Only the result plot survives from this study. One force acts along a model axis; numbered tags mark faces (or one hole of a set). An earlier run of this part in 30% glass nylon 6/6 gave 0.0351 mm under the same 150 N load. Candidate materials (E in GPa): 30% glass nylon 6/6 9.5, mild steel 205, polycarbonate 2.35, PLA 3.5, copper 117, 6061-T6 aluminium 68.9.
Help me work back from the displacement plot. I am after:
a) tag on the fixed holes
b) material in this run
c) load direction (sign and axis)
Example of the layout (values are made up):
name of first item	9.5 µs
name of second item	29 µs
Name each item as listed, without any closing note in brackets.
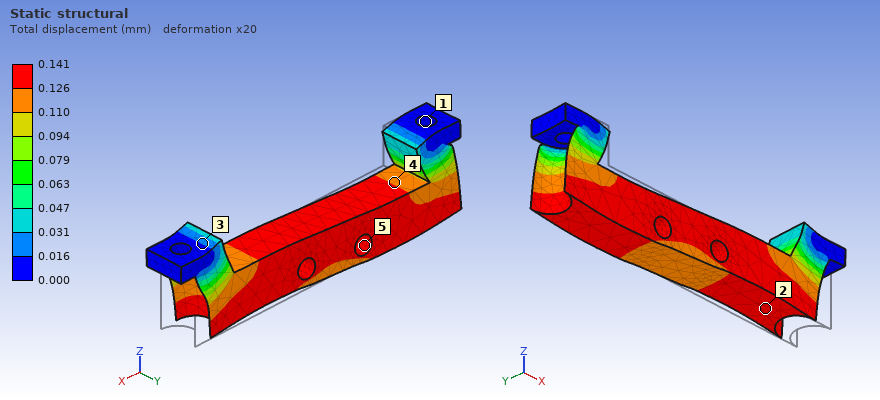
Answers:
tag on the fixed holes	1
material in this run	polycarbonate
load direction	-X
